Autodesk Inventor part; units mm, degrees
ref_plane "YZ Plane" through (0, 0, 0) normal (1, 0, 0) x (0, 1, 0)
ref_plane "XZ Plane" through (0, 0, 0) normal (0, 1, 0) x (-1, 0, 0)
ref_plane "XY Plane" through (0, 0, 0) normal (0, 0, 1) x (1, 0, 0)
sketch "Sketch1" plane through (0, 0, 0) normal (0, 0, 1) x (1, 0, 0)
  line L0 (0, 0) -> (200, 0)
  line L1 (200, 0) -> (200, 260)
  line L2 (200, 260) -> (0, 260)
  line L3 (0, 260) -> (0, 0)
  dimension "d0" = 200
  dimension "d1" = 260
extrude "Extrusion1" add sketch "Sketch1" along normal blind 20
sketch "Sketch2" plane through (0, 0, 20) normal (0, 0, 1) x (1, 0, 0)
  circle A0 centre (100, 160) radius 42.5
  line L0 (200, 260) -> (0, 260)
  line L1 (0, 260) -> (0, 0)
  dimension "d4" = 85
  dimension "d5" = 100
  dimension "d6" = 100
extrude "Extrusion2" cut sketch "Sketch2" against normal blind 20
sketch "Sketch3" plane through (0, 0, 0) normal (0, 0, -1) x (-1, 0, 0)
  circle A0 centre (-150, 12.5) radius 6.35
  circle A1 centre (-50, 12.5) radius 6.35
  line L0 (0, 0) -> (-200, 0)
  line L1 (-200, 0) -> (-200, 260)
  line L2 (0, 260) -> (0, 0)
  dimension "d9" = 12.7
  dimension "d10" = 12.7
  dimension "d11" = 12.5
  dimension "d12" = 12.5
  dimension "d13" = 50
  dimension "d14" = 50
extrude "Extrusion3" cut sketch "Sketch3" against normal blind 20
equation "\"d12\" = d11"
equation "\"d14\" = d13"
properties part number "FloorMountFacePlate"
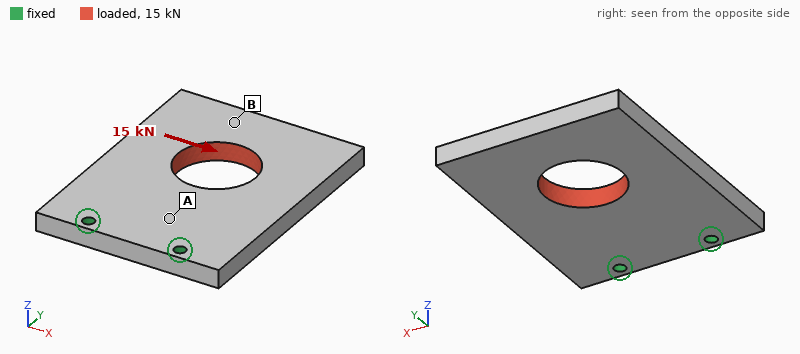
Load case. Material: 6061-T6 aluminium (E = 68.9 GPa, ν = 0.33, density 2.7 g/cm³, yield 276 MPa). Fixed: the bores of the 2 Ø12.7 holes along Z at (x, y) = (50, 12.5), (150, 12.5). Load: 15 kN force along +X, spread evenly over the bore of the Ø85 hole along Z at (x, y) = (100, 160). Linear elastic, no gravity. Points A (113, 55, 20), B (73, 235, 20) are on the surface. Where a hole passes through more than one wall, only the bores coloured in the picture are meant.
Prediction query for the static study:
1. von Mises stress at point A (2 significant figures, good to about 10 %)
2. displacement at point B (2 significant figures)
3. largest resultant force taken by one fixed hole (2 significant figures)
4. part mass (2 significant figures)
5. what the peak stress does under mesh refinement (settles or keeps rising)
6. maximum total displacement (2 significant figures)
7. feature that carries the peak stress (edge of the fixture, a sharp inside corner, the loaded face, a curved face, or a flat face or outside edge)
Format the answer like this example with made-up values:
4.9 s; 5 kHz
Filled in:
17 MPa; 0.14 mm; 22 kN; 2.5 kg; keeps rising; 0.15 mm; edge of the fixture
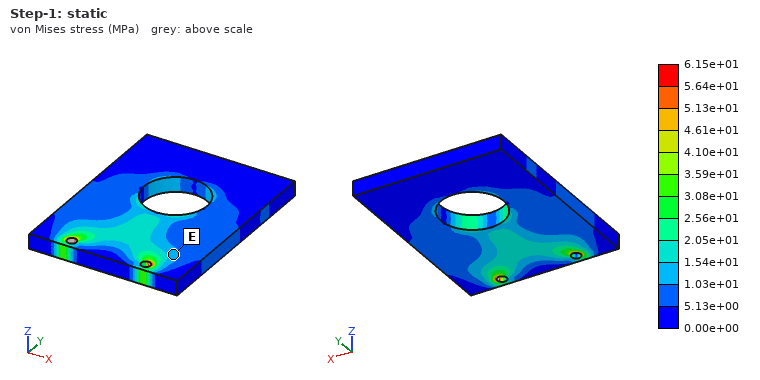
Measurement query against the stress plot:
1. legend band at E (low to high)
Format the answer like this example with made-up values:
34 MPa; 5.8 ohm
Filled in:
1.03e+01 to 1.54e+01 MPa
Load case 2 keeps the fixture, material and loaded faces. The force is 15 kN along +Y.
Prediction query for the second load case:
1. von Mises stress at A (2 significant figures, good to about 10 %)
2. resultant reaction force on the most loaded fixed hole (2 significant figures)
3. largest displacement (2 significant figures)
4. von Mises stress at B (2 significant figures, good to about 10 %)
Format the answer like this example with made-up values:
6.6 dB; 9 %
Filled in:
2.7 MPa; 7.5 kN; 20 µm; 2.8 MPa
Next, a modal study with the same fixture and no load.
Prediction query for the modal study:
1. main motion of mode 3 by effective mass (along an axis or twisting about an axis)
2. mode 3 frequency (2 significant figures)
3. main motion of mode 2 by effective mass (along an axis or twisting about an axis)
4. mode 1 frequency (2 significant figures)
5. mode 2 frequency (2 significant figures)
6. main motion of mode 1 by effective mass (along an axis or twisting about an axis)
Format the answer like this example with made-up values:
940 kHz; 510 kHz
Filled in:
along X; 1300 Hz; twisting about Y; 250 Hz; 650 Hz; along Z
